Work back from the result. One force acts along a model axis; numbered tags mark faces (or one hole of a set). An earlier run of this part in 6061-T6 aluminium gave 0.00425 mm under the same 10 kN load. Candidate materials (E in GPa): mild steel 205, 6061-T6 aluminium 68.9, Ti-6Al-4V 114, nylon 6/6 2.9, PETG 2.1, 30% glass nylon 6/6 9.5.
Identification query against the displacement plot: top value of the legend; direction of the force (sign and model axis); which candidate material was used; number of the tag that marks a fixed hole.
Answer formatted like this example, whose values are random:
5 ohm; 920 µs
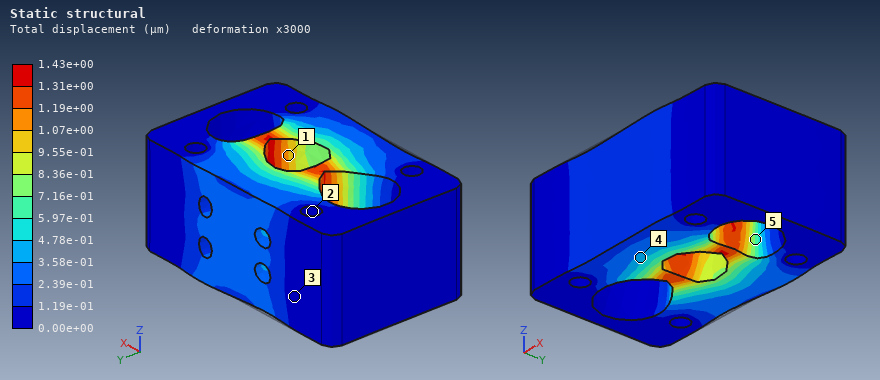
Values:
1.43e+00 µm; +X; mild steel; 2
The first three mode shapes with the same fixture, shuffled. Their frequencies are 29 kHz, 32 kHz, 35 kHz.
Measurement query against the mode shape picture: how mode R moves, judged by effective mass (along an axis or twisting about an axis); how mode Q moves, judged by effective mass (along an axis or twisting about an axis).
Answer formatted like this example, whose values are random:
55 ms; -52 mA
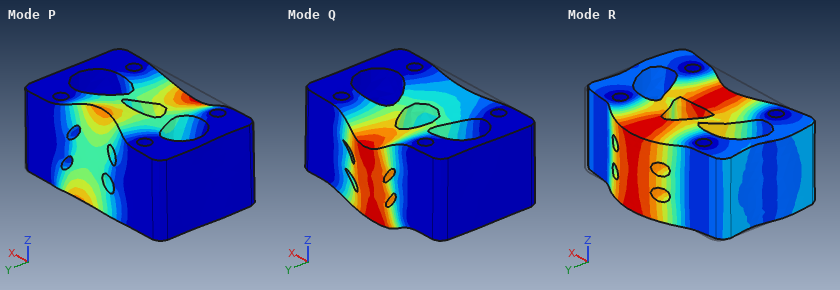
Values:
along Y; along Z
